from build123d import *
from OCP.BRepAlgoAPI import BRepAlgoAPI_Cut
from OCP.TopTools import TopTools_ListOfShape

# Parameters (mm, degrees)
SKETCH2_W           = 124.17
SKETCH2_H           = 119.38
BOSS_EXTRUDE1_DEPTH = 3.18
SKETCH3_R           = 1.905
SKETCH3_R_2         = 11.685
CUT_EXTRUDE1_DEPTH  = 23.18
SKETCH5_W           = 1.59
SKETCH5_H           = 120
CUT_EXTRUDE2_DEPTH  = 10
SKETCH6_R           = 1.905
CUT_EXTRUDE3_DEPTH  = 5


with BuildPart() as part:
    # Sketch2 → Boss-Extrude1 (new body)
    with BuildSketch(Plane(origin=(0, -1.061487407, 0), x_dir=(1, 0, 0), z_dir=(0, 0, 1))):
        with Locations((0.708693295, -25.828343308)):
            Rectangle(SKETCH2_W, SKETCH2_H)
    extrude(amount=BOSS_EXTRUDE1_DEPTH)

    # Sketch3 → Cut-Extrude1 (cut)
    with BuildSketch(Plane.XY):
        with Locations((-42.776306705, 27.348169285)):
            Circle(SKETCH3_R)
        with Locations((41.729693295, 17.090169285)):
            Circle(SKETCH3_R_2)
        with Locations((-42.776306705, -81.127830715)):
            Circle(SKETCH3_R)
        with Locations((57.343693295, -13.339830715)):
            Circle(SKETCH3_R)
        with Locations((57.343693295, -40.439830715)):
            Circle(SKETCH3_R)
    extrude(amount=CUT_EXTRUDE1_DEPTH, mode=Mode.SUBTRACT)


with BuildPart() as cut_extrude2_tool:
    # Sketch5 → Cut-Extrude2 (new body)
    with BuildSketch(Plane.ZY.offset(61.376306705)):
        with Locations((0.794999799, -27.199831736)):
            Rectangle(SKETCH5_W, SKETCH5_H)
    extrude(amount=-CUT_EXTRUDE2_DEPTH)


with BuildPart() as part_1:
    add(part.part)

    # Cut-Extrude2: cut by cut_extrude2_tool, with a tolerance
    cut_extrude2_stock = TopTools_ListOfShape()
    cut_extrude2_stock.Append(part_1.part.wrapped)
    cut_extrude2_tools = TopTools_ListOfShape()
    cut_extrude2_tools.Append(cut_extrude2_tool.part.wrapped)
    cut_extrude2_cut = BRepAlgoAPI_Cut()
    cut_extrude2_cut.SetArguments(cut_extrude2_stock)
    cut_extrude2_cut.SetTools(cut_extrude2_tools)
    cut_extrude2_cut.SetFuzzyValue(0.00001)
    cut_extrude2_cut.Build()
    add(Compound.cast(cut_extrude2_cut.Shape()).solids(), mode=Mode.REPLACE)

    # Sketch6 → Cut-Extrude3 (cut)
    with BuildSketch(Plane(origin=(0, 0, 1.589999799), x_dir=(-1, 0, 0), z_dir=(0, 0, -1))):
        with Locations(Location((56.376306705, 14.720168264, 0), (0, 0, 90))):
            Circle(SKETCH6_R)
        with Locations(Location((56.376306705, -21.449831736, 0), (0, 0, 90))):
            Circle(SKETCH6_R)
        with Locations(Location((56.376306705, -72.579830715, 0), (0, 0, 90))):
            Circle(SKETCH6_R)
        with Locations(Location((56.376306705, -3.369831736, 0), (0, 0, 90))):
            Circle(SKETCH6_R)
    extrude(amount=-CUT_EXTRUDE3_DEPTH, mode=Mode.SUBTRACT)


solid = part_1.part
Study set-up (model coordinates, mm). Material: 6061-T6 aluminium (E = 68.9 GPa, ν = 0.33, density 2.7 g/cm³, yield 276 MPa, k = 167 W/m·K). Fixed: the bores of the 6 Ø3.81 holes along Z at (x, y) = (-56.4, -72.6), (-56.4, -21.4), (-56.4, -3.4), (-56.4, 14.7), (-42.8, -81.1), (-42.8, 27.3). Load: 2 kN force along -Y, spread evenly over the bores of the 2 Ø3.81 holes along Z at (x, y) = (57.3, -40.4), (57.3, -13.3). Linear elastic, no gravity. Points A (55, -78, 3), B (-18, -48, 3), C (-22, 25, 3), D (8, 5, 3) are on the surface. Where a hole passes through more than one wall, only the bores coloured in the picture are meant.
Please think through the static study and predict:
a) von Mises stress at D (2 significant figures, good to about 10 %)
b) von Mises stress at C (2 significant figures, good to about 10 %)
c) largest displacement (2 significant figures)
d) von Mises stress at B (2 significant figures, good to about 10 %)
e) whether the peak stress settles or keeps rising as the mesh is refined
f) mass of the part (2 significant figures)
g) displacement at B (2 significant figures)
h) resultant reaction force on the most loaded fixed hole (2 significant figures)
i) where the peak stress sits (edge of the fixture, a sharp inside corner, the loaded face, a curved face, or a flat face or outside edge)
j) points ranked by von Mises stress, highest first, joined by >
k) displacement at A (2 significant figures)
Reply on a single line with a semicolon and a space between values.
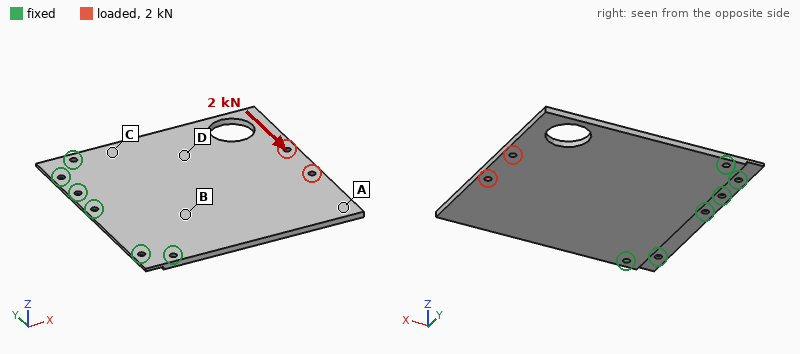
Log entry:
14 MPa; 21 MPa; 58 µm; 11 MPa; keeps rising; 120 g; 11 µm; 1.7 kN; edge of the fixture; C > D > B > A; 53 µm
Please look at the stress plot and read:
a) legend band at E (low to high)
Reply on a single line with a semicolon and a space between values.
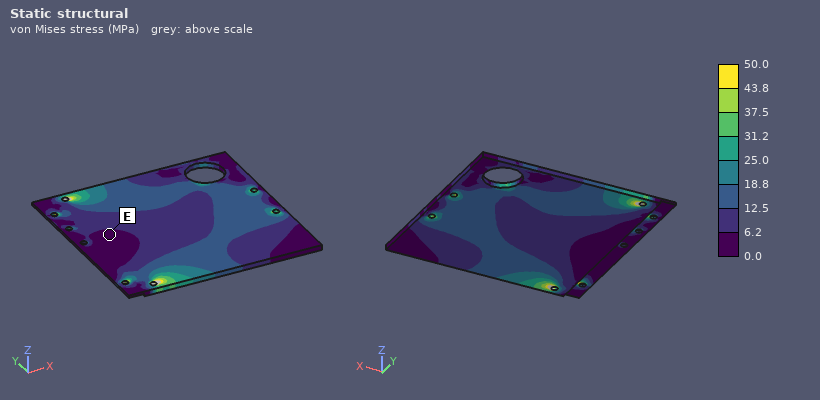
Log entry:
0.0 to 6.2 MPa
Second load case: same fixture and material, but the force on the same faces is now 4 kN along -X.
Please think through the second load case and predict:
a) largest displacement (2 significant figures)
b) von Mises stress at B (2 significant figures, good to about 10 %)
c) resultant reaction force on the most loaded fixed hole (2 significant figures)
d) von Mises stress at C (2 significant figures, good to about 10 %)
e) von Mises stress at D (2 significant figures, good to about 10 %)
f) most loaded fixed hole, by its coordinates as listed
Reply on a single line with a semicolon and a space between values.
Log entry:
93 µm; 9.1 MPa; 1.1 kN; 12 MPa; 14 MPa; (-42.8, -81.1)
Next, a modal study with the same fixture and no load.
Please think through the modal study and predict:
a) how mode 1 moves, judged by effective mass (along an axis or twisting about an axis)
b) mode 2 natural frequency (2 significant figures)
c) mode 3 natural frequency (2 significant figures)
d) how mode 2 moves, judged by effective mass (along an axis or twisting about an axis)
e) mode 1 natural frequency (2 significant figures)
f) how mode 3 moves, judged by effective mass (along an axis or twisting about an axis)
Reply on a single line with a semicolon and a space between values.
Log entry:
along Z; 550 Hz; 1200 Hz; twisting about X; 200 Hz; along Z
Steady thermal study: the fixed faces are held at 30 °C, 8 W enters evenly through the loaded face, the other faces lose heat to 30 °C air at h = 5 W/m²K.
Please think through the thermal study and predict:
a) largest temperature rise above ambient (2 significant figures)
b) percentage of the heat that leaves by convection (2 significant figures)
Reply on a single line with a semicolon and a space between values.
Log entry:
18 K; 13 %
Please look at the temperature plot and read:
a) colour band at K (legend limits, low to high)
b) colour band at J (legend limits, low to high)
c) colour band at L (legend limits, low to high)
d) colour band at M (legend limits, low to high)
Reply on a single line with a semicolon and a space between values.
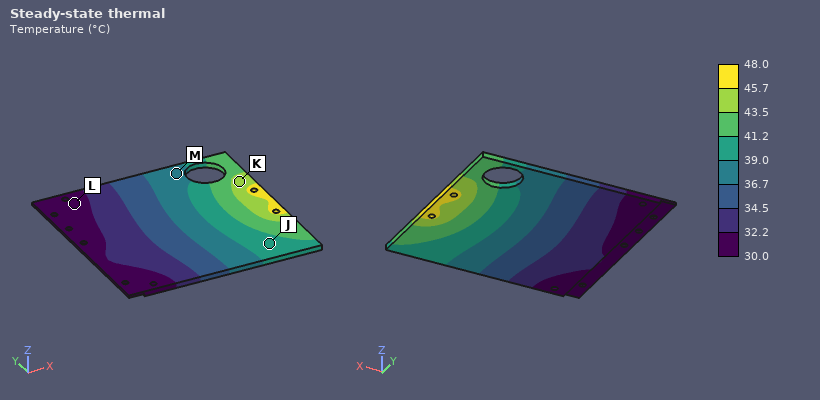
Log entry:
43.5 to 45.7 °C; 39.0 to 41.2 °C; 30.0 to 32.2 °C; 36.7 to 39.0 °C
